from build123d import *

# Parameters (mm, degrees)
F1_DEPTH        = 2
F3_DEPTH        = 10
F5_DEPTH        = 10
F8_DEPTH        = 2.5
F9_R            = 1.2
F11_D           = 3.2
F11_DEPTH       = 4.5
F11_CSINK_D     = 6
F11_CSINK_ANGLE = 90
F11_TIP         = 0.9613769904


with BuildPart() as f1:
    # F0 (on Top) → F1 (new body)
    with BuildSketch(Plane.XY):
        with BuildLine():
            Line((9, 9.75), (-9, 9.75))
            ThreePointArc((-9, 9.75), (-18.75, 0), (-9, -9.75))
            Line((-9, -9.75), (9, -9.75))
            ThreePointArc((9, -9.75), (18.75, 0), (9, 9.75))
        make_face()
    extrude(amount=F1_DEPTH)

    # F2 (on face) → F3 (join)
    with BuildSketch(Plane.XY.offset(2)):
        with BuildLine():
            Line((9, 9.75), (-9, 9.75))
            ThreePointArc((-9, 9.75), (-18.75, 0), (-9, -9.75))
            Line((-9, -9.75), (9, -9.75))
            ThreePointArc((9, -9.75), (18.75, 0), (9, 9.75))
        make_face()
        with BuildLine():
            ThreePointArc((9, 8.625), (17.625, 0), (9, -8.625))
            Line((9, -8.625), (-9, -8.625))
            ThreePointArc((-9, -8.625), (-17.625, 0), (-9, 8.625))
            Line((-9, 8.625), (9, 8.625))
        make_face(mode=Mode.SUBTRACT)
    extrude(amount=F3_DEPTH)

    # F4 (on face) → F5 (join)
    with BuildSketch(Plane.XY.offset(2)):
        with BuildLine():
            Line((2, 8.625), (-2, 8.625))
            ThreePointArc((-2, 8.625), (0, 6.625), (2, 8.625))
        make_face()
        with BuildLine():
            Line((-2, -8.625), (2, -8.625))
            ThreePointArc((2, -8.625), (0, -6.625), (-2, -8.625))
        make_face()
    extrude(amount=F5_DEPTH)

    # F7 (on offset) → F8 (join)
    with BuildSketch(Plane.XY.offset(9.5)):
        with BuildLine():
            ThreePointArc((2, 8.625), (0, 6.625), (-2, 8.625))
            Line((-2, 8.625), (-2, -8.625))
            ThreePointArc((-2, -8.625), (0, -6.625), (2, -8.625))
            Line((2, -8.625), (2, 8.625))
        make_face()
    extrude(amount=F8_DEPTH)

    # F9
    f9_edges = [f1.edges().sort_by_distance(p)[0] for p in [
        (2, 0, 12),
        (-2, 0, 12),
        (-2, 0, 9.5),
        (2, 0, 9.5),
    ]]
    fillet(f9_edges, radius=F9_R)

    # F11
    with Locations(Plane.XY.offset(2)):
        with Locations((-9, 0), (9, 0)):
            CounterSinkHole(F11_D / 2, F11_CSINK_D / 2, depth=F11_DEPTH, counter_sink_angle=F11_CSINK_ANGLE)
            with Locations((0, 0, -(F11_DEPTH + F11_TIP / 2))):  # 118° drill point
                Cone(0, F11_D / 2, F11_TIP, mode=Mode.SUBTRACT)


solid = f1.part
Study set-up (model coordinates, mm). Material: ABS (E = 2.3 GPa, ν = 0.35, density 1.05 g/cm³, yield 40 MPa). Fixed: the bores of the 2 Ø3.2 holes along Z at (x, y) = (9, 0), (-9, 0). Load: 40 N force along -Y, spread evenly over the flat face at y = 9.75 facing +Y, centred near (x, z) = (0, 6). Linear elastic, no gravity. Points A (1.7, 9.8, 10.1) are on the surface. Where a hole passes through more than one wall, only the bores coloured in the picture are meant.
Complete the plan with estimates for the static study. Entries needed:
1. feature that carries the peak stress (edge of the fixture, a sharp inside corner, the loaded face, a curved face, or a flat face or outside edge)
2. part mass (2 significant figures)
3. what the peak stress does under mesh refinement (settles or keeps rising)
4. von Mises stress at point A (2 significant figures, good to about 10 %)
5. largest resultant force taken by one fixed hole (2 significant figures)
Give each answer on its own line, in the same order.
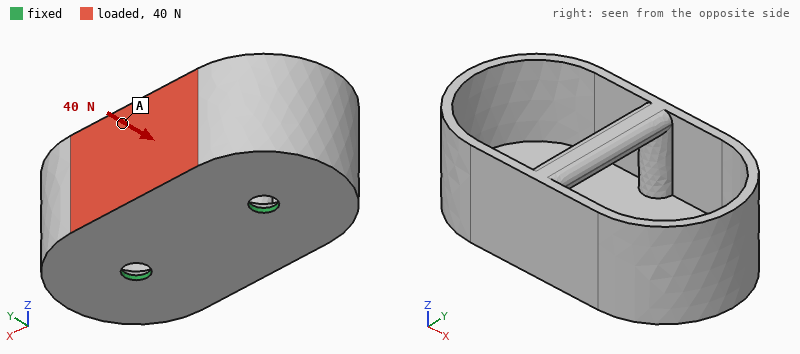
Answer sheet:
edge of the fixture
2.7 g
keeps rising
3.9 MPa
20 N
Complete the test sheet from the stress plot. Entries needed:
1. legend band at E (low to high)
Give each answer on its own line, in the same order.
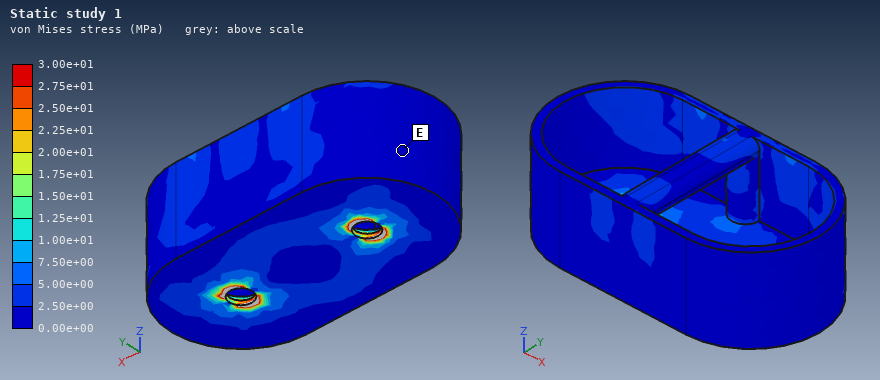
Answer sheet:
0.00e+00 to 2.50e+00 MPa
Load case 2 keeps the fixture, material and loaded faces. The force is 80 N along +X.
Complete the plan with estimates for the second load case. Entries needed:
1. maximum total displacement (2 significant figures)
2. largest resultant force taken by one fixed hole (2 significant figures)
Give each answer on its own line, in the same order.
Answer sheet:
0.21 mm
61 N
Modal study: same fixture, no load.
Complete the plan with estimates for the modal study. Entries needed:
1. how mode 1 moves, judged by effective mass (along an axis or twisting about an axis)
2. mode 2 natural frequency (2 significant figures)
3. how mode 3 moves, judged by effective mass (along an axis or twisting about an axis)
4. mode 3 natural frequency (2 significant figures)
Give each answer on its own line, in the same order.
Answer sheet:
along Y
2500 Hz
along X
2600 Hz
